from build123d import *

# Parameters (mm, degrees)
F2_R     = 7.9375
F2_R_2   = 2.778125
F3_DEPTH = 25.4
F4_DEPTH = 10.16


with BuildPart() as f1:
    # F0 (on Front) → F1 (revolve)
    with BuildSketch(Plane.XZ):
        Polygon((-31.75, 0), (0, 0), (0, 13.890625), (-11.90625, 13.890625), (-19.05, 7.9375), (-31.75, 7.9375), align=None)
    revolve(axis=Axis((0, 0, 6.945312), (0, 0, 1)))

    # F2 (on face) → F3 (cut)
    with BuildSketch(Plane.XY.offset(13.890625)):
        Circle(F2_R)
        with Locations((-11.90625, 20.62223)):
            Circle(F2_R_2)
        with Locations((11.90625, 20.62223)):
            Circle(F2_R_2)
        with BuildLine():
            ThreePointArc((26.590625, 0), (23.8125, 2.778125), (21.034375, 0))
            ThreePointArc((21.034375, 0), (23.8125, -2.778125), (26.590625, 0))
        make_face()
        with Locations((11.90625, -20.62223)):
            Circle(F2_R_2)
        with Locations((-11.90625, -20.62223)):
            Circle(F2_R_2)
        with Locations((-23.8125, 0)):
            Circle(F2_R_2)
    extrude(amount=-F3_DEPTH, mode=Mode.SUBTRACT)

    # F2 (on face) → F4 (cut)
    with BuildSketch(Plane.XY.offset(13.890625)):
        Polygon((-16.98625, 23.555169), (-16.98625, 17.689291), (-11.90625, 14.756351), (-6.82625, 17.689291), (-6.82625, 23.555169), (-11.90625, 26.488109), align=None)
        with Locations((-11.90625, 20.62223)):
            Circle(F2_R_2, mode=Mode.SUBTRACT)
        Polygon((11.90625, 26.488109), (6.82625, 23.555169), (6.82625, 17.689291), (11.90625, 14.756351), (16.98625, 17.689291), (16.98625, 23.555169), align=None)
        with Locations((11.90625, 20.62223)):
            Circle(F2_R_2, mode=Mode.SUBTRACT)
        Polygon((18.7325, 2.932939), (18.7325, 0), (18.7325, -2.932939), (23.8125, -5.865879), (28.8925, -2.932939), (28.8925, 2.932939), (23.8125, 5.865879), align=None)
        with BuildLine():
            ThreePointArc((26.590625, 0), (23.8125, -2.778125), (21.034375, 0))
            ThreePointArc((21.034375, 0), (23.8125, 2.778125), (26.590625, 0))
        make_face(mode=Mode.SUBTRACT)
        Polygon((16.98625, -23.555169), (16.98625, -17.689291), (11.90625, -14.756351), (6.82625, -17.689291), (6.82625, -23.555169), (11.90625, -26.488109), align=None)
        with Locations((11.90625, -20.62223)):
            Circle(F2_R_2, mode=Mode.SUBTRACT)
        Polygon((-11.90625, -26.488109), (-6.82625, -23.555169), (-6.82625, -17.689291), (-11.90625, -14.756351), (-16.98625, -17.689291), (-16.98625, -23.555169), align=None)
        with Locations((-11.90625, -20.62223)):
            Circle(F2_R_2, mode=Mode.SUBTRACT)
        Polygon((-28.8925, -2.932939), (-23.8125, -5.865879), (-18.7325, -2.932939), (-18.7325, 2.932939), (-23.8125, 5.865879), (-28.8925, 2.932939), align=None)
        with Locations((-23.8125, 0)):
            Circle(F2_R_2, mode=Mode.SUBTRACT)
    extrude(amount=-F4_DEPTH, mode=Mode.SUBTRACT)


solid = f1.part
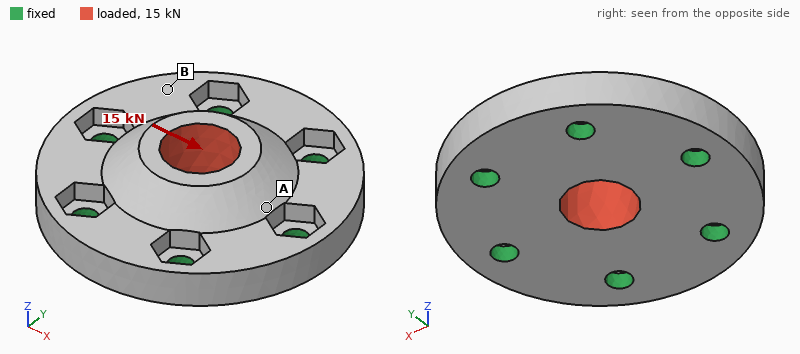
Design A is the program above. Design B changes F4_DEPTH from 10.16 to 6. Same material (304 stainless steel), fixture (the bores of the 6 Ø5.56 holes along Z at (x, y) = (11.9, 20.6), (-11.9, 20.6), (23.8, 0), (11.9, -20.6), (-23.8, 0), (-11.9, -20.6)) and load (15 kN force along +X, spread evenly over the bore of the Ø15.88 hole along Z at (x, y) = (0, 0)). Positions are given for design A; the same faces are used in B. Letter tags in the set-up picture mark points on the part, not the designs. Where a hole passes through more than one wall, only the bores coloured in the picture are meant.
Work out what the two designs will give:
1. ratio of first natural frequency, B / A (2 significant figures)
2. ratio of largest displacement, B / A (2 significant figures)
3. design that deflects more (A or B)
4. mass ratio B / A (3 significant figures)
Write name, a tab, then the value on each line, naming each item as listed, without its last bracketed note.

ratio of first natural frequency, B / A	1.2
ratio of largest displacement, B / A	0.67
design that deflects more	A
mass ratio B / A	1.07
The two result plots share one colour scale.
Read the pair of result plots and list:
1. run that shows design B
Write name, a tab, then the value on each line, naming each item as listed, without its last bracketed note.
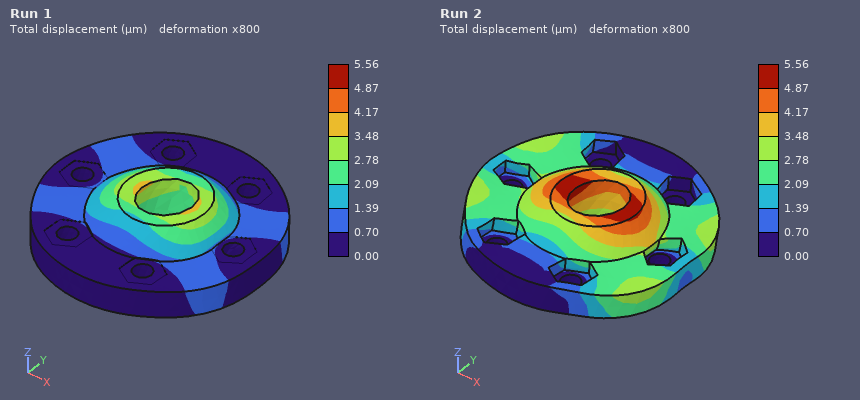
run that shows design B	Run 1
